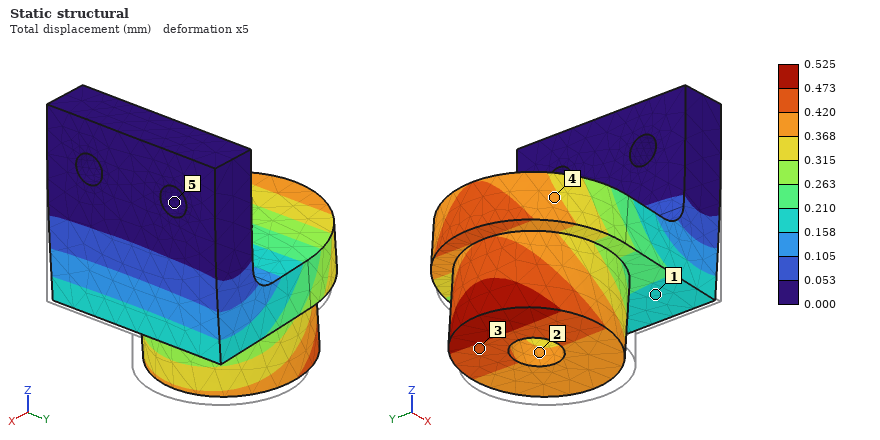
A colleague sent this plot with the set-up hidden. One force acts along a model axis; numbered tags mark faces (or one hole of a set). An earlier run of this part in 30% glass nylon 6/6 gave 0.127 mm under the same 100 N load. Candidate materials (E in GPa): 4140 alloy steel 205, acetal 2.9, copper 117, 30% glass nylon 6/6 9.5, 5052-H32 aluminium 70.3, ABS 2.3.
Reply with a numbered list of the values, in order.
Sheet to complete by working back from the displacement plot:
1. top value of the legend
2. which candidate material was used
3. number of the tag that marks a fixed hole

1. 0.525 mm
2. ABS
3. 5
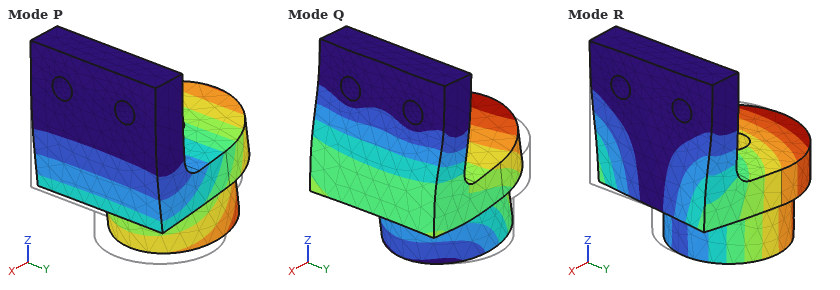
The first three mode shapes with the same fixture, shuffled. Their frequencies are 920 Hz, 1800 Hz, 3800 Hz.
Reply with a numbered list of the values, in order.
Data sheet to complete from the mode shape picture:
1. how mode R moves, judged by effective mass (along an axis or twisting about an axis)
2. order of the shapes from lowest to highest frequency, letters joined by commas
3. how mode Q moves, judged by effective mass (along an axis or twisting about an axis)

1. along Y
2. P, R, Q
3. along X
